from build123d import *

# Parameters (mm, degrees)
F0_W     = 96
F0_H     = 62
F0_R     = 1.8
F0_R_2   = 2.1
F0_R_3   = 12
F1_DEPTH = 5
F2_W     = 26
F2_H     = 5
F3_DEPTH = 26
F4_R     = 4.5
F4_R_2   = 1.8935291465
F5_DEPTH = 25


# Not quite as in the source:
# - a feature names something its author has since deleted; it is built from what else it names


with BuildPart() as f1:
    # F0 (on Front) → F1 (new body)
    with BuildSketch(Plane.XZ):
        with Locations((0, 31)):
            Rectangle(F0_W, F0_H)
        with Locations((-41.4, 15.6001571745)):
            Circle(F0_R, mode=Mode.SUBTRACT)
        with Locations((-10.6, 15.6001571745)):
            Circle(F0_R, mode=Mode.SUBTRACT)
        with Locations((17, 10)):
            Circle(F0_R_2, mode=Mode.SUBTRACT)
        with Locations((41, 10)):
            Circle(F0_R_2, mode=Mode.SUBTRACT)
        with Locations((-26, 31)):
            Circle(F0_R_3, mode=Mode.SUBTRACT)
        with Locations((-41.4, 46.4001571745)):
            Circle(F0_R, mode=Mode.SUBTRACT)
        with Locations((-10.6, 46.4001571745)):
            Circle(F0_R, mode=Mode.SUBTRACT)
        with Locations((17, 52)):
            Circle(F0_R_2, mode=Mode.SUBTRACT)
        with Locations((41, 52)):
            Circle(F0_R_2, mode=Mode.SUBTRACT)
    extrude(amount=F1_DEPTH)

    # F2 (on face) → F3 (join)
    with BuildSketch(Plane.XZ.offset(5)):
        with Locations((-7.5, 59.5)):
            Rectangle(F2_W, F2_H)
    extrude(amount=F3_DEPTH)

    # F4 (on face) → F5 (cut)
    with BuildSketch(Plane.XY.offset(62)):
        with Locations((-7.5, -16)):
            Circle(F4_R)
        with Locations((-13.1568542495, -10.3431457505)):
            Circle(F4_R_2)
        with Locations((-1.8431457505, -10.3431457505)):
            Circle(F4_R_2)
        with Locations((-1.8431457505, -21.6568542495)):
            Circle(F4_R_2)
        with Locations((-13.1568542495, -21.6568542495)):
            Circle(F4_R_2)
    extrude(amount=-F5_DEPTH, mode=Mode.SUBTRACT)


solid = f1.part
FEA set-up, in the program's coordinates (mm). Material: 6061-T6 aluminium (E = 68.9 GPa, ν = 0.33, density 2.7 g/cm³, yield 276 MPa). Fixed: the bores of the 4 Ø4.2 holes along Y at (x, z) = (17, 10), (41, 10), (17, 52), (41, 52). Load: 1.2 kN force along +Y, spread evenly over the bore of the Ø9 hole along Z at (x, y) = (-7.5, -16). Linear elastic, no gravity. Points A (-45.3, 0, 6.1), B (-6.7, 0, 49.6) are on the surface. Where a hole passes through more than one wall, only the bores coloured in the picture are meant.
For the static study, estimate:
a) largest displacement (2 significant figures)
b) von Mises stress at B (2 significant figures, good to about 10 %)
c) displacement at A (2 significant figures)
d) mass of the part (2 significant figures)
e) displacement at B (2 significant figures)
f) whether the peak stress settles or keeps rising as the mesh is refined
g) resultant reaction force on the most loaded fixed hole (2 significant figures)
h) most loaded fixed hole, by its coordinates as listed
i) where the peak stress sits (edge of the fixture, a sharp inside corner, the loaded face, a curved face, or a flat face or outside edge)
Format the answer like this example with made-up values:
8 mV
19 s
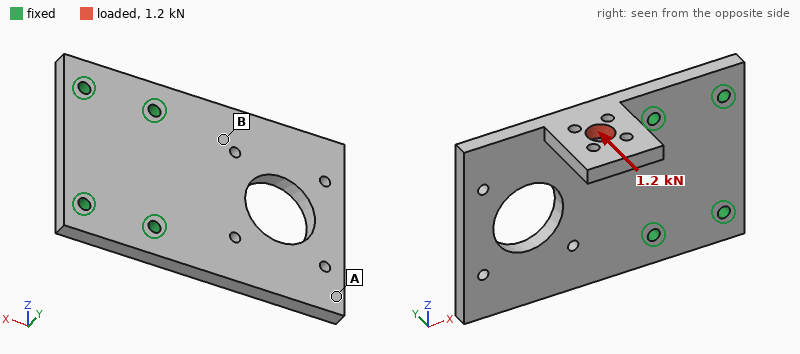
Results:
0.79 mm
57 MPa
0.31 mm
81 g
0.21 mm
keeps rising
1.6 kN
(17, 52)
edge of the fixture
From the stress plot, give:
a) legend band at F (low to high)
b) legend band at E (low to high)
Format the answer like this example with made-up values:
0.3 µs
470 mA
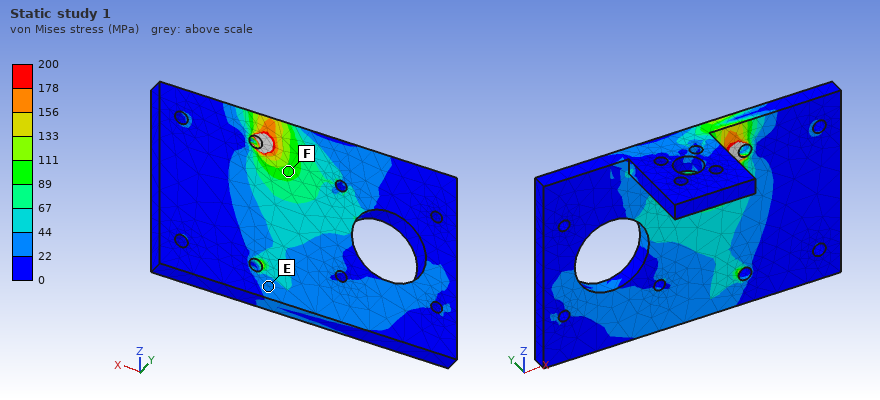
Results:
89 to 111 MPa
22 to 44 MPa
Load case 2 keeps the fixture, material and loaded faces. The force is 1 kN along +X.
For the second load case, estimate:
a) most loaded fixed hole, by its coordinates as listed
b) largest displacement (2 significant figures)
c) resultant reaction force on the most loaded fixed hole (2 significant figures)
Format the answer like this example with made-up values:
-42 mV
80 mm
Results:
(17, 52)
0.52 mm
950 N
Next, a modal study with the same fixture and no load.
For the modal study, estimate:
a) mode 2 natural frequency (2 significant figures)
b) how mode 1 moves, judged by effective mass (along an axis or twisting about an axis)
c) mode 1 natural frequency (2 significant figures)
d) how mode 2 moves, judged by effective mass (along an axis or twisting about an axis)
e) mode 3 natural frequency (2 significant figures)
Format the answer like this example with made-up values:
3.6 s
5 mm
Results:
2000 Hz
along Y
990 Hz
twisting about X
3400 Hz
